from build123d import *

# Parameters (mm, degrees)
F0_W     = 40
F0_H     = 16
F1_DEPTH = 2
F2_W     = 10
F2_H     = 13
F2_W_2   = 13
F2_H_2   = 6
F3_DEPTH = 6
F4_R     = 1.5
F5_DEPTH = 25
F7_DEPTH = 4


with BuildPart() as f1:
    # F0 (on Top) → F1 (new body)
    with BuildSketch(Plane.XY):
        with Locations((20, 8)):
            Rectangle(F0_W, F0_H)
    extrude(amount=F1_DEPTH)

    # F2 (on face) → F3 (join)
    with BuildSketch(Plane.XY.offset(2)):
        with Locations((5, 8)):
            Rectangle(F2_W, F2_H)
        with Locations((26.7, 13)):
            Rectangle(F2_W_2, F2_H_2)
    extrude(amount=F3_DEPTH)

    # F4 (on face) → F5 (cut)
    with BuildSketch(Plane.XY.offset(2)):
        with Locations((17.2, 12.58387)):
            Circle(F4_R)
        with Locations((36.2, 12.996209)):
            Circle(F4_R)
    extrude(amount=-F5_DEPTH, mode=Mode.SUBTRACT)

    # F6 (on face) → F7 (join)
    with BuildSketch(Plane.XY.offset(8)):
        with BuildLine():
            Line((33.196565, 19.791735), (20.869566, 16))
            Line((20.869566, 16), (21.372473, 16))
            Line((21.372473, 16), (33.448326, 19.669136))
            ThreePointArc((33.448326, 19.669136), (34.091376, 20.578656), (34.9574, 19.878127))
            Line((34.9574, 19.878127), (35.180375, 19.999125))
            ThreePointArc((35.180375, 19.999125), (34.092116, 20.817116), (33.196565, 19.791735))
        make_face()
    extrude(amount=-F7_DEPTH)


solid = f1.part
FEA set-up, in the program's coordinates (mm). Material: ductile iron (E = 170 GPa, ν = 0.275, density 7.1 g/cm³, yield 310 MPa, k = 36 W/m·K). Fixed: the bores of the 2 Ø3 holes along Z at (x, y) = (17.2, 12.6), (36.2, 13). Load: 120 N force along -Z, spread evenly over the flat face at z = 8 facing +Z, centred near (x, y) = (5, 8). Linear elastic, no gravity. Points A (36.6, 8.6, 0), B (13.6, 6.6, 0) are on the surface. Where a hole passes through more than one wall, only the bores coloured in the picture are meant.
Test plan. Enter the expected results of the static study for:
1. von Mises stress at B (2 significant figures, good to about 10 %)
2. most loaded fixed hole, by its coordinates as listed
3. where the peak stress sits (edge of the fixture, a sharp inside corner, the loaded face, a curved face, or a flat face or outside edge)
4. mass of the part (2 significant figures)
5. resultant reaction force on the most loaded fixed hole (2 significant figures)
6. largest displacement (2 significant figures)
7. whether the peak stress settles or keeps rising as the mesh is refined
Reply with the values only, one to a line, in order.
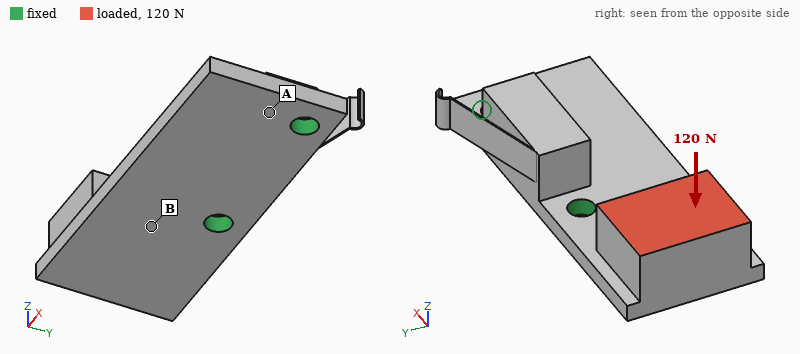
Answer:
76 MPa
(17.2, 12.6)
edge of the fixture
18 g
140 N
87 µm
keeps rising
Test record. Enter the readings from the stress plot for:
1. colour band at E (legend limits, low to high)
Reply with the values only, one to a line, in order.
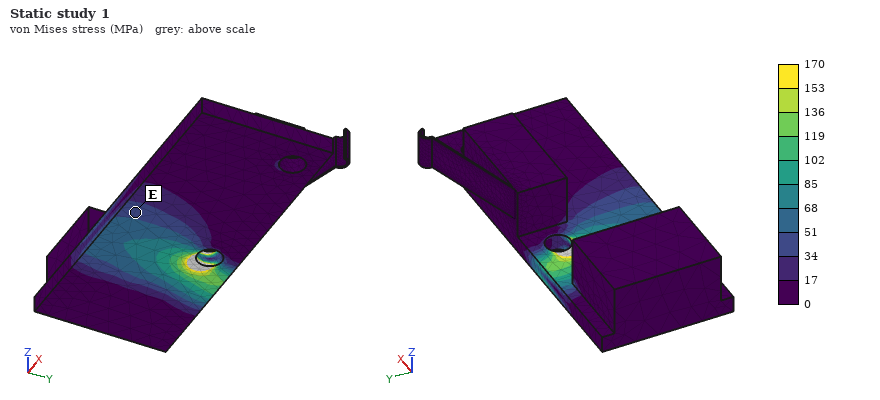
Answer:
34 to 51 MPa
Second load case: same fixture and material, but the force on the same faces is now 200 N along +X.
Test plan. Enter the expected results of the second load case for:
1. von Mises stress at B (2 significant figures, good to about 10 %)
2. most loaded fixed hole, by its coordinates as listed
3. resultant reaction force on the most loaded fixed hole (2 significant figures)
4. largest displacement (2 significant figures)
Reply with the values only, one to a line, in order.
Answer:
100 MPa
(17.2, 12.6)
150 N
0.10 mm
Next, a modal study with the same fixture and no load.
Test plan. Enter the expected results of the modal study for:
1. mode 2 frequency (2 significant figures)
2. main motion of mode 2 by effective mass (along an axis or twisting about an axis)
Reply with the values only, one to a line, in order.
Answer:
2600 Hz
along Z
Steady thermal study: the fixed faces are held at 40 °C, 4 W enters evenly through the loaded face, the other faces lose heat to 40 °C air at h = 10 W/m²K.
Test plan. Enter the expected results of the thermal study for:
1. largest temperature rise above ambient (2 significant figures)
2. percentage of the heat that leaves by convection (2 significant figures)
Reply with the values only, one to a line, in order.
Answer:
43 K
7.2 %
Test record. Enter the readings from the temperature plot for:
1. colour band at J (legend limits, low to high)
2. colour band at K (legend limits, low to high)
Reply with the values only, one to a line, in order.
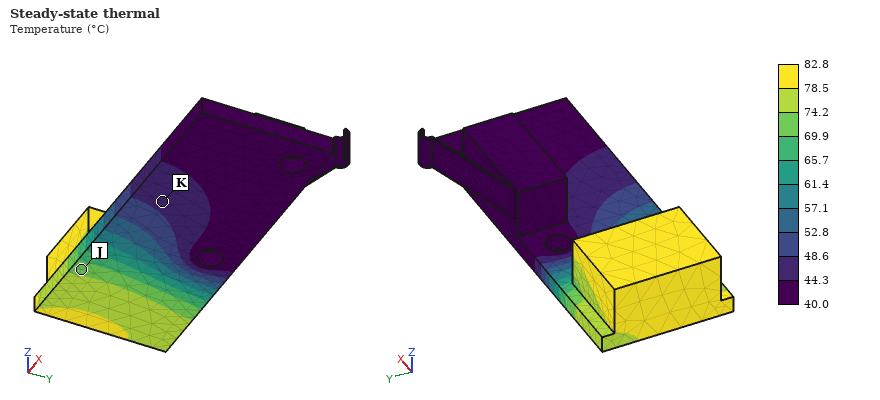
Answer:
69.9 to 74.2 °C
44.3 to 48.6 °C
